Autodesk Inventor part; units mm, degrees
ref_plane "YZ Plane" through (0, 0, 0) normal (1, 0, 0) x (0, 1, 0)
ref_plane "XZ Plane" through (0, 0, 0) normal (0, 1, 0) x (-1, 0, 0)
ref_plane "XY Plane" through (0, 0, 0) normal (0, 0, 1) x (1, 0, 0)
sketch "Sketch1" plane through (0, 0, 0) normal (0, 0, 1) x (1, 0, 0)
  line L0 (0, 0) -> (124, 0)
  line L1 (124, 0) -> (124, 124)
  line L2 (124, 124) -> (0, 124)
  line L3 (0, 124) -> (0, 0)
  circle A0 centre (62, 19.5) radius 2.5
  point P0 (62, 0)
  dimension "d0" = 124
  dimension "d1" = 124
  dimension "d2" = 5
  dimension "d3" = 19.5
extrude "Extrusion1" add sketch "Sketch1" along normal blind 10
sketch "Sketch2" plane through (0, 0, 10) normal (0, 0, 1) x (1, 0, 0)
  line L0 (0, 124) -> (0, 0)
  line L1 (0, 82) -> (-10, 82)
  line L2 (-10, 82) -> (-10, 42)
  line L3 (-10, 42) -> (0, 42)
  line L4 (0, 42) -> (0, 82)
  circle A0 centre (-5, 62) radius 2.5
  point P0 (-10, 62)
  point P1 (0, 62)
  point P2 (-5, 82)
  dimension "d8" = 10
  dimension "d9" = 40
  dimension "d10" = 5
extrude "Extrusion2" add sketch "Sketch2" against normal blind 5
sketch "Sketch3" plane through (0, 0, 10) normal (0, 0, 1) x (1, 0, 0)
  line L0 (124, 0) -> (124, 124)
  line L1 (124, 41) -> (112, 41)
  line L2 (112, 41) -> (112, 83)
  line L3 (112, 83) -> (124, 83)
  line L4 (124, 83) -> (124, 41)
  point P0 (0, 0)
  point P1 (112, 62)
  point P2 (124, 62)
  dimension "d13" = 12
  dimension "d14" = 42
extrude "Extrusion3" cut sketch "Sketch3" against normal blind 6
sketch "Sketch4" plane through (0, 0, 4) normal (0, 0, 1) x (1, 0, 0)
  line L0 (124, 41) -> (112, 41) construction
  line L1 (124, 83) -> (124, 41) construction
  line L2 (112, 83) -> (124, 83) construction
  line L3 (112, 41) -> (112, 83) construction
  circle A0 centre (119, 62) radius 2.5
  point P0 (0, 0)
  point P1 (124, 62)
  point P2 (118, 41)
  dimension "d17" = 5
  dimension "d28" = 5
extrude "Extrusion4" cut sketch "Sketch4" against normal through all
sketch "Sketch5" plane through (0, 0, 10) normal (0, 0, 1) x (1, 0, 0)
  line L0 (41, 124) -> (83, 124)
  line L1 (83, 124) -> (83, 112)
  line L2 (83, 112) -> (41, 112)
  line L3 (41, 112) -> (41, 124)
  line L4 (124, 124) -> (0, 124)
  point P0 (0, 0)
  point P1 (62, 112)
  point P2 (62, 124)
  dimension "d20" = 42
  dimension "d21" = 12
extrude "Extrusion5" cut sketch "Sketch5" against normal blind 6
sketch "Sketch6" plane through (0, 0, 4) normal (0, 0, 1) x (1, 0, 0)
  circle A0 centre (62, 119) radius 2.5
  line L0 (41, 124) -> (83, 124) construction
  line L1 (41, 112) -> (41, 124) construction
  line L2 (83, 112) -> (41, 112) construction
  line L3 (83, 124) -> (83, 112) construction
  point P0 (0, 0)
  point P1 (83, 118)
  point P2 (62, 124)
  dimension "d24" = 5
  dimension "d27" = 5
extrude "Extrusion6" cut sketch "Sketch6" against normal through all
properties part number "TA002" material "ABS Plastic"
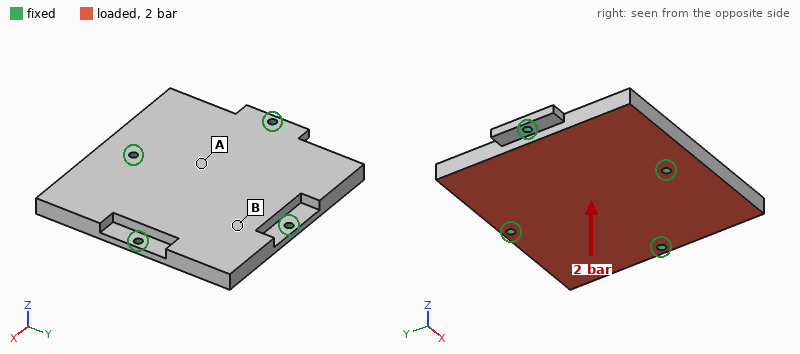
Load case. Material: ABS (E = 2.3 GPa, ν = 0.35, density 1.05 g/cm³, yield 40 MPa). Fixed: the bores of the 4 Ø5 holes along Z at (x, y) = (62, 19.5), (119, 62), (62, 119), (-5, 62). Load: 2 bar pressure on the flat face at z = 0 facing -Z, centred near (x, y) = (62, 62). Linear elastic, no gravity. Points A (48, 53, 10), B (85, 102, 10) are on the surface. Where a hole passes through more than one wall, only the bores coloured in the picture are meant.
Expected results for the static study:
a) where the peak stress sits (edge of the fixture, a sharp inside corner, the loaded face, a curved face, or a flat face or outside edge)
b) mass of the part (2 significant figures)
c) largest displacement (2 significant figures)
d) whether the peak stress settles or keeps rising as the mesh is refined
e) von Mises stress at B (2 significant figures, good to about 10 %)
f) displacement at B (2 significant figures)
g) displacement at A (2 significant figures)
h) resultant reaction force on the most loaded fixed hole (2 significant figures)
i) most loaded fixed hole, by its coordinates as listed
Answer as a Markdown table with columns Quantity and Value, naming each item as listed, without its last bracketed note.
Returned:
| Quantity | Value |
|---|---|
| where the peak stress sits | edge of the fixture |
| mass of the part | 160 g |
| largest displacement | 1.1 mm |
| whether the peak stress settles or keeps rising as the mesh is refined | keeps rising |
| von Mises stress at B | 8.4 MPa |
| displacement at B | 0.50 mm |
| displacement at A | 0.34 mm |
| resultant reaction force on the most loaded fixed hole | 1.1 kN |
| most loaded fixed hole, by its coordinates as listed | (62, 19.5) |
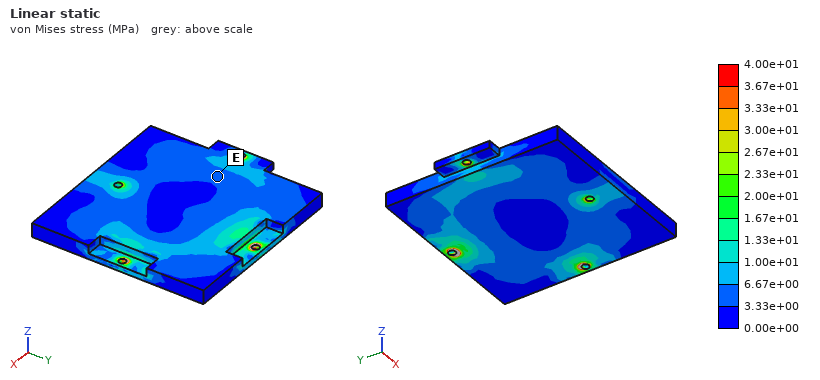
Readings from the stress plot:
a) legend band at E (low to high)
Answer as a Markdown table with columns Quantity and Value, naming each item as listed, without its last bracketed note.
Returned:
| Quantity | Value |
|---|---|
| legend band at E | 3.33e+00 to 6.67e+00 MPa |
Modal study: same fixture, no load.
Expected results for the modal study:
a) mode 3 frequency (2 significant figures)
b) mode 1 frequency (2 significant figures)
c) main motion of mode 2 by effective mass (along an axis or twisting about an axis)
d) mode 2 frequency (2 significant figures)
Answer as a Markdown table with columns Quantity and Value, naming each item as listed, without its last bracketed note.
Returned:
| Quantity | Value |
|---|---|
| mode 3 frequency | 910 Hz |
| mode 1 frequency | 740 Hz |
| main motion of mode 2 by effective mass | along Z |
| mode 2 frequency | 840 Hz |
